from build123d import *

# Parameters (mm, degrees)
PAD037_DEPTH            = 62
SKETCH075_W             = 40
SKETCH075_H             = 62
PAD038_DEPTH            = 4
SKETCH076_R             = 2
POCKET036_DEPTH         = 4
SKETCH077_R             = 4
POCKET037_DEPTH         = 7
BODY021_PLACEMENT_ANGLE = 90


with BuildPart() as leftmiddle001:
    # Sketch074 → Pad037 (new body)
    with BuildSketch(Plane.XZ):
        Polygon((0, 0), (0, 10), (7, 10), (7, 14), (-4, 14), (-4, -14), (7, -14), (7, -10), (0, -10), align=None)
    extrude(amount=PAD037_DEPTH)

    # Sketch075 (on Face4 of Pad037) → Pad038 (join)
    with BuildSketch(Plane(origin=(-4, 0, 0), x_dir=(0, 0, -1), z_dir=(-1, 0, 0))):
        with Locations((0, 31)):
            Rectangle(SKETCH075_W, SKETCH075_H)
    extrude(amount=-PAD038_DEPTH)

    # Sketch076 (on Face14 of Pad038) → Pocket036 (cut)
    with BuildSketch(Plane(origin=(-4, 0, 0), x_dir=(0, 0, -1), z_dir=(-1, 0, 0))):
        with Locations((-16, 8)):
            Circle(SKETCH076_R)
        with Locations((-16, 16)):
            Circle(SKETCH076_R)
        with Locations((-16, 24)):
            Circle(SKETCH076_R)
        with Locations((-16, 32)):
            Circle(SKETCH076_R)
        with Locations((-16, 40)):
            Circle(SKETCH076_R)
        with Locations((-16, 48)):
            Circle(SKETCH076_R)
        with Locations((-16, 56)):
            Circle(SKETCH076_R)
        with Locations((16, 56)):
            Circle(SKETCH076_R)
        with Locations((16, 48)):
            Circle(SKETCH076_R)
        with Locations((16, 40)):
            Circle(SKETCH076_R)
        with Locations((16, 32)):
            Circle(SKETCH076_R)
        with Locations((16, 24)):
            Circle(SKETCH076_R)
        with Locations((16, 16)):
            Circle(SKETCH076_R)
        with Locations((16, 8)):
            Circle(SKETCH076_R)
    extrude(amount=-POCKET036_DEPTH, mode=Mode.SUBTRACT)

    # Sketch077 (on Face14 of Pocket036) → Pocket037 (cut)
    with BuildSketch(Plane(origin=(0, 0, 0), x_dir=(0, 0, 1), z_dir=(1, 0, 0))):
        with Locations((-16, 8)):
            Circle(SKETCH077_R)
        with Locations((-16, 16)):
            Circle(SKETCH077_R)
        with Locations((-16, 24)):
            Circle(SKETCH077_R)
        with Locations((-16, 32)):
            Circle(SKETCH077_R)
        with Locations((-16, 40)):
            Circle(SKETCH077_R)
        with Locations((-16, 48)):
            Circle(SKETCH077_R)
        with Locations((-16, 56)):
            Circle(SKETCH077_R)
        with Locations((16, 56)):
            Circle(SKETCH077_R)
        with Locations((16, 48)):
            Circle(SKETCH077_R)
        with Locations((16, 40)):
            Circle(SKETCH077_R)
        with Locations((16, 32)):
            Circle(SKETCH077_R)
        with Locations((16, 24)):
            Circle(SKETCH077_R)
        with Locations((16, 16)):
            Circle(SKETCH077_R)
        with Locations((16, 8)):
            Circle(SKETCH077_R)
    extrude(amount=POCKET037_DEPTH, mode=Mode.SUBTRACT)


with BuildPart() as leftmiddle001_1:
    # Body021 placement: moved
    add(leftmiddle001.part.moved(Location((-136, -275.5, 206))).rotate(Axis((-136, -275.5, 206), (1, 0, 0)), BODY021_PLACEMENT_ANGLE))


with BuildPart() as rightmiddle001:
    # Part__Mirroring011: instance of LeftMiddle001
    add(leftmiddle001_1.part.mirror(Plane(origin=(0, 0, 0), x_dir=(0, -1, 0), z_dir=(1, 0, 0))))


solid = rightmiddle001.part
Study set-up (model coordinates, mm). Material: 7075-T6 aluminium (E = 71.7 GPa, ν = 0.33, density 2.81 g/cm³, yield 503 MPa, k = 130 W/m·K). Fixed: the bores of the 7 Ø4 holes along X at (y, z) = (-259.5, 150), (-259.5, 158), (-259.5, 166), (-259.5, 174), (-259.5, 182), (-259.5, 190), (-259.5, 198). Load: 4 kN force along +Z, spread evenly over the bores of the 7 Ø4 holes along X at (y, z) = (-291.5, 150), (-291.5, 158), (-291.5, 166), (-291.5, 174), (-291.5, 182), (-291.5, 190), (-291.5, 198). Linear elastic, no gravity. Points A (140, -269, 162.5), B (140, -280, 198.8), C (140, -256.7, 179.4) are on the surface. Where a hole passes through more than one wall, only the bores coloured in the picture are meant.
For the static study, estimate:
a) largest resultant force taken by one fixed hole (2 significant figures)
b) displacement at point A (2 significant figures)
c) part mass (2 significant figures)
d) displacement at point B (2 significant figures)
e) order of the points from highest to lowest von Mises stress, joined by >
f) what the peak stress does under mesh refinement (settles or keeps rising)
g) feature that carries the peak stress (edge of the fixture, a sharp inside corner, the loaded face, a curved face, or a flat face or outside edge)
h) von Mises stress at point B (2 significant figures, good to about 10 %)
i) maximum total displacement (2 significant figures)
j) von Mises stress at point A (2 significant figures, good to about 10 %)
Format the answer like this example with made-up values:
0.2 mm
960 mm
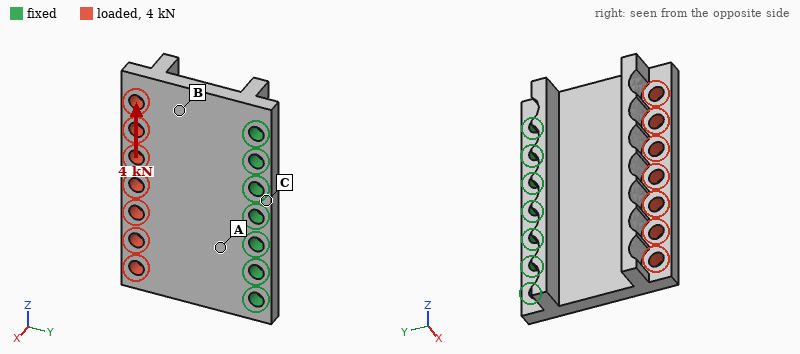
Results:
2.1 kN
6.5 µm
33 g
21 µm
A > B > C
keeps rising
edge of the fixture
21 MPa
42 µm
38 MPa
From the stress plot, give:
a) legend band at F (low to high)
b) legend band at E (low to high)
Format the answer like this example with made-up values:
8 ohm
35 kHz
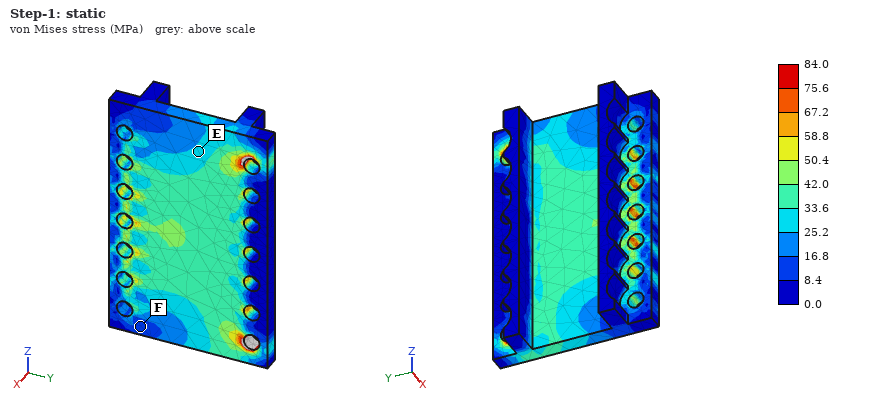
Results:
8.4 to 16.8 MPa
25.2 to 33.6 MPa
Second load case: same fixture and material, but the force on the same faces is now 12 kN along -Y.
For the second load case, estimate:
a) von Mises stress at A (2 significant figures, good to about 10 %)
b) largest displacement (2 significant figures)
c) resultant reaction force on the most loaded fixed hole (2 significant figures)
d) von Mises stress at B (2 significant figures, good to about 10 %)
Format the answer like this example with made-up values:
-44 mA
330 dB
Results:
51 MPa
29 µm
2.2 kN
43 MPa
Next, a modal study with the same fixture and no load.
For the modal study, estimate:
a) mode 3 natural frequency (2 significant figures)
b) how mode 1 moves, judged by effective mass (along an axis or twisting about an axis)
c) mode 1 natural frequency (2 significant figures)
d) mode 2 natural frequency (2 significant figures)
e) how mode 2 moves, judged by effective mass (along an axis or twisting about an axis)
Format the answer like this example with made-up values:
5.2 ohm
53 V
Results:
12 kHz
along X
2600 Hz
4000 Hz
twisting about Y
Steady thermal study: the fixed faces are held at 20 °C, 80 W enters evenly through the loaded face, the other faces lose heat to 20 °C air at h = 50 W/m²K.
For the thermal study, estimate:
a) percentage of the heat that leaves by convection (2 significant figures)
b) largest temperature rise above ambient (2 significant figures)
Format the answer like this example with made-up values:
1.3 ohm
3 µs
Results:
15 %
76 K
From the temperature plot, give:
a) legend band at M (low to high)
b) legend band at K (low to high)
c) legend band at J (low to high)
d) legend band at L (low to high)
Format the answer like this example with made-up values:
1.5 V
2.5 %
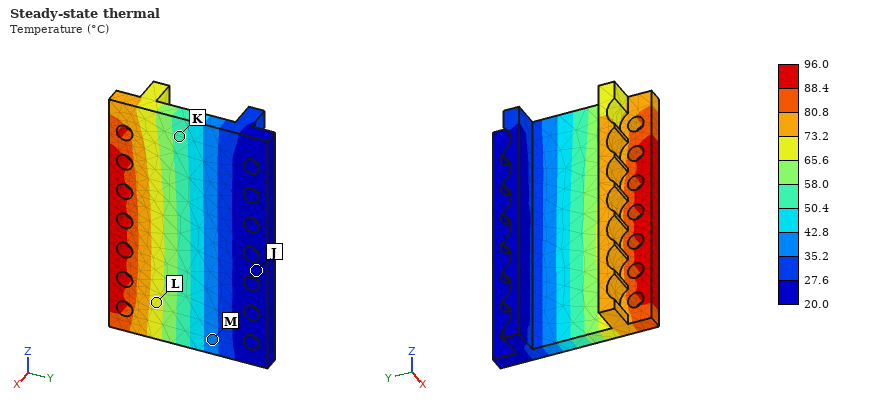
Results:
35.2 to 42.8 °C
50.4 to 58.0 °C
20.0 to 27.6 °C
65.6 to 73.2 °C
